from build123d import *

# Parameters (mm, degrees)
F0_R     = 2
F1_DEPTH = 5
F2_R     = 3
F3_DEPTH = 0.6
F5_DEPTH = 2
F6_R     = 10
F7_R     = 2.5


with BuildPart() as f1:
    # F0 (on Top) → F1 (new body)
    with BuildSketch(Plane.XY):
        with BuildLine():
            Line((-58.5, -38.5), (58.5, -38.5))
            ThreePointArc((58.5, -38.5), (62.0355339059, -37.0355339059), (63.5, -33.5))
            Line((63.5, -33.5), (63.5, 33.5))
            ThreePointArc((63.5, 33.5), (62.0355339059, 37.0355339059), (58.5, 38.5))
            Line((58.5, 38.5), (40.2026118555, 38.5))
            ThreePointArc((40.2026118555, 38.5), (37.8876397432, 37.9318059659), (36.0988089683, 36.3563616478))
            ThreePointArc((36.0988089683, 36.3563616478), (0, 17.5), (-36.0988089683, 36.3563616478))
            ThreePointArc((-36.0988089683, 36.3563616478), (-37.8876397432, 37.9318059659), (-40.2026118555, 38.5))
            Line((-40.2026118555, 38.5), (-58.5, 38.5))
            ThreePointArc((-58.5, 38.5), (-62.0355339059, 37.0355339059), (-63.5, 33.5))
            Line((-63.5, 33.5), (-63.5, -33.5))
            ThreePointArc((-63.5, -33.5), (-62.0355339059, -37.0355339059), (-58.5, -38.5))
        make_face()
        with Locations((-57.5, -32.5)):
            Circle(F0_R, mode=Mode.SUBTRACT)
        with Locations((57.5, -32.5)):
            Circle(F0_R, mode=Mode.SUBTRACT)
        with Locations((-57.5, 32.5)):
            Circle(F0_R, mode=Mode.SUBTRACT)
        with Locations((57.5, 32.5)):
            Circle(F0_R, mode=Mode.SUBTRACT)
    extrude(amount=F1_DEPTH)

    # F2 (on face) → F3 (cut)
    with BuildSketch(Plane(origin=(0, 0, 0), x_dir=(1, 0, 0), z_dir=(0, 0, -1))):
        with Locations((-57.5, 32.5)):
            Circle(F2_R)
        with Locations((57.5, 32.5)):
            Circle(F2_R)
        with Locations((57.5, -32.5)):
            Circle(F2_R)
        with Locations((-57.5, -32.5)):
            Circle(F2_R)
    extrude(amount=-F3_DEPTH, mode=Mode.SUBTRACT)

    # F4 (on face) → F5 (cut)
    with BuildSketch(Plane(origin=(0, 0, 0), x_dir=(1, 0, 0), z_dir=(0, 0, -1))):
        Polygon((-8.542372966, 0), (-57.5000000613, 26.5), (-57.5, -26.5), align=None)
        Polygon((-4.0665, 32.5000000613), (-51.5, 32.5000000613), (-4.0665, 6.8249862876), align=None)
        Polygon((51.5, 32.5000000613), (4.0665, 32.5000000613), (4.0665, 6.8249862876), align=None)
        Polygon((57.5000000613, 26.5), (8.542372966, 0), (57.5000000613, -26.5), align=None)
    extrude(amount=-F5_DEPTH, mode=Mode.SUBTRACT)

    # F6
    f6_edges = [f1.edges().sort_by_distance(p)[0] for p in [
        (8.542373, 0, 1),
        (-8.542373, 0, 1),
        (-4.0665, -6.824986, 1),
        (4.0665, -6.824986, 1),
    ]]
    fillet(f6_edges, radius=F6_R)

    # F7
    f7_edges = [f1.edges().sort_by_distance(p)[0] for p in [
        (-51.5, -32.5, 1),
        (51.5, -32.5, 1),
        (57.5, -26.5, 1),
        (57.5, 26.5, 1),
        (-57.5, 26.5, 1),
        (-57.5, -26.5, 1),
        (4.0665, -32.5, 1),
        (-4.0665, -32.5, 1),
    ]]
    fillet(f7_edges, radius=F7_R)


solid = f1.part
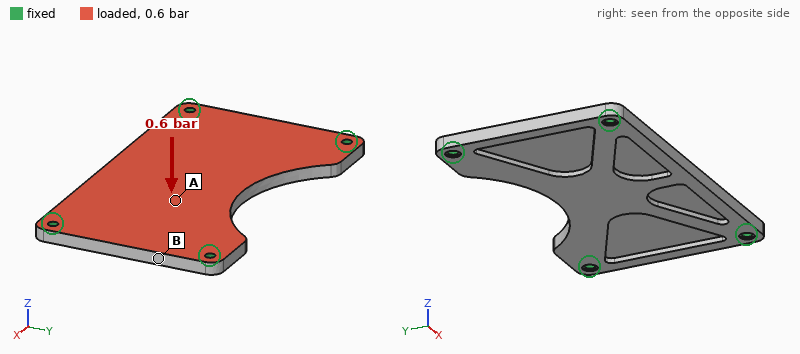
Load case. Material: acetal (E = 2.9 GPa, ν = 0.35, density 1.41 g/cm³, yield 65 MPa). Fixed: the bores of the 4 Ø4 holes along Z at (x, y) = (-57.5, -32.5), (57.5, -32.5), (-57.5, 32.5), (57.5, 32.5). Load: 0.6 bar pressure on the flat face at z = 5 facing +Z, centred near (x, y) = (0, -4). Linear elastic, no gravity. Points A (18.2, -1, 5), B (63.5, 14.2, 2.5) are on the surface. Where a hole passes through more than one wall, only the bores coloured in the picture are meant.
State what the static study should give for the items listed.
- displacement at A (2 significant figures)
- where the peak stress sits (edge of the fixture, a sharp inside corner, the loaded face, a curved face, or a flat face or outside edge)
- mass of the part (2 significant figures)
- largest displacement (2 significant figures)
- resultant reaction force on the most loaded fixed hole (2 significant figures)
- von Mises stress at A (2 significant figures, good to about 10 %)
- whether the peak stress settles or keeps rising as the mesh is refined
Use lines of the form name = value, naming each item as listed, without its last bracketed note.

displacement at A = 1.5 mm
where the peak stress sits = edge of the fixture
mass of the part = 51 g
largest displacement = 1.7 mm
resultant reaction force on the most loaded fixed hole = 160 N
von Mises stress at A = 7.2 MPa
whether the peak stress settles or keeps rising as the mesh is refined = keeps rising
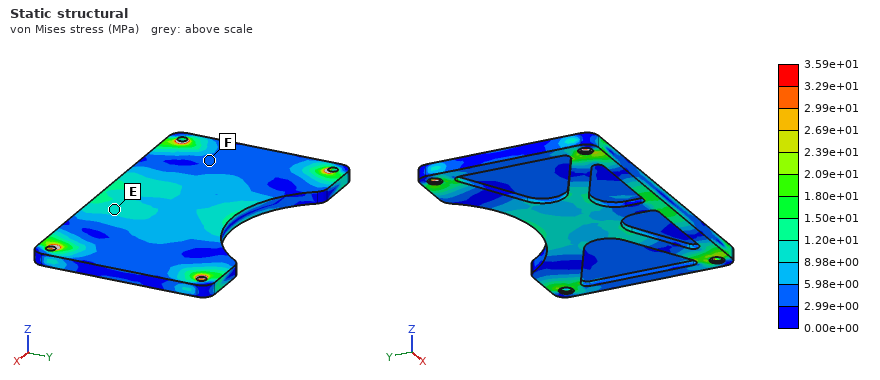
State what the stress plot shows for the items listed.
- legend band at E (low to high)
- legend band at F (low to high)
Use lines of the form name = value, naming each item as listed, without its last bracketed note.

legend band at E = 8.98e+00 to 1.20e+01 MPa
legend band at F = 2.99e+00 to 5.98e+00 MPa
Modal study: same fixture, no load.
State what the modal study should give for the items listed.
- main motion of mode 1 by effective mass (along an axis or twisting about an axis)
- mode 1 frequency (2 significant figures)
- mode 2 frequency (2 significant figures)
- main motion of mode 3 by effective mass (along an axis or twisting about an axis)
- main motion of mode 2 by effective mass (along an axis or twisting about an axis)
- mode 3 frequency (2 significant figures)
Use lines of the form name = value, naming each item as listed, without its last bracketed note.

main motion of mode 1 by effective mass = along Z
mode 1 frequency = 440 Hz
mode 2 frequency = 810 Hz
main motion of mode 3 by effective mass = twisting about Y
main motion of mode 2 by effective mass = twisting about X
mode 3 frequency = 1100 Hz
